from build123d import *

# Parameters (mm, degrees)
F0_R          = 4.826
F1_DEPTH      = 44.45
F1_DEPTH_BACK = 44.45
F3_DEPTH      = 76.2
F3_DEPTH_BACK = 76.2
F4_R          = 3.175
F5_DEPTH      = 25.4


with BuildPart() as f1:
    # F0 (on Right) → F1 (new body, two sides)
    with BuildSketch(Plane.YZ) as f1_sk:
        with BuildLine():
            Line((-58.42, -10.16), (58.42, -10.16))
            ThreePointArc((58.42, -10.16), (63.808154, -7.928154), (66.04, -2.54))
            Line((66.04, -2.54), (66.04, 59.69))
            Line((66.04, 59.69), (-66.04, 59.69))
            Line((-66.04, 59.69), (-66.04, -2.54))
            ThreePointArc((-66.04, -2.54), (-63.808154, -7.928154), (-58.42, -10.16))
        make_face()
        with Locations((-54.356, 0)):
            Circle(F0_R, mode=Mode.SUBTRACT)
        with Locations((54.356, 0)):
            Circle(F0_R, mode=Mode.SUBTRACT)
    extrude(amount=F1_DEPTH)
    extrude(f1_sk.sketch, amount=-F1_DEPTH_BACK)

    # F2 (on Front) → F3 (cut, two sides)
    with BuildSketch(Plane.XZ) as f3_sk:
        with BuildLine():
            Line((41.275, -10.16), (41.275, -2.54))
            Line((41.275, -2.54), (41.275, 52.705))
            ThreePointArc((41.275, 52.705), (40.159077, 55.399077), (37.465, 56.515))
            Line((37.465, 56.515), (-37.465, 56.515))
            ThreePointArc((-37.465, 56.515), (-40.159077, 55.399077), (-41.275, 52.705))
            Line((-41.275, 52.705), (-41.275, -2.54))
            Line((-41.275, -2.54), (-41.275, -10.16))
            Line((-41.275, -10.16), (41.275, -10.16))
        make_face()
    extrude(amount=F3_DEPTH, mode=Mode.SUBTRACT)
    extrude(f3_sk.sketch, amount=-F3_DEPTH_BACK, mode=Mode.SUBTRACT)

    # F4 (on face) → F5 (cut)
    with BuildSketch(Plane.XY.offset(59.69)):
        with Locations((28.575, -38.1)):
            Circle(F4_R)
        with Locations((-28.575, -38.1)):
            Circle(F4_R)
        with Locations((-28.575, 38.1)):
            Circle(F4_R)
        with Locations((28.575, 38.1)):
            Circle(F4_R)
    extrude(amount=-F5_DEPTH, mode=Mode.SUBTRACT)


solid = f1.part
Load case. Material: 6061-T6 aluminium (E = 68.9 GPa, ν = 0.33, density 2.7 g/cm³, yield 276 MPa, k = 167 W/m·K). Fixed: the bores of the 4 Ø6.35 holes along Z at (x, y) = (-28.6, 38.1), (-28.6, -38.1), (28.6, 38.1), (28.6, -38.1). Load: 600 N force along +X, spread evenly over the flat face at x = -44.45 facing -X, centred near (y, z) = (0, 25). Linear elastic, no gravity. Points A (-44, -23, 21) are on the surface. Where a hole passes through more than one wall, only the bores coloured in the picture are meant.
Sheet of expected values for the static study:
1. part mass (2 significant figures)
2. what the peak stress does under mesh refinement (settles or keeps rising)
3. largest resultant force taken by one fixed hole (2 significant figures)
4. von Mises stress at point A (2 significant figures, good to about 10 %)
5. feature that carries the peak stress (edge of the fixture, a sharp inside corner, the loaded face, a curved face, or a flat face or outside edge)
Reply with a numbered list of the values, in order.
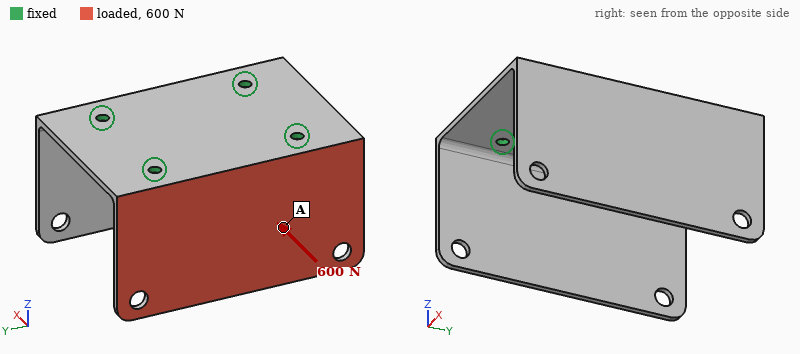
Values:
1. 250 g
2. keeps rising
3. 230 N
4. 16 MPa
5. edge of the fixture
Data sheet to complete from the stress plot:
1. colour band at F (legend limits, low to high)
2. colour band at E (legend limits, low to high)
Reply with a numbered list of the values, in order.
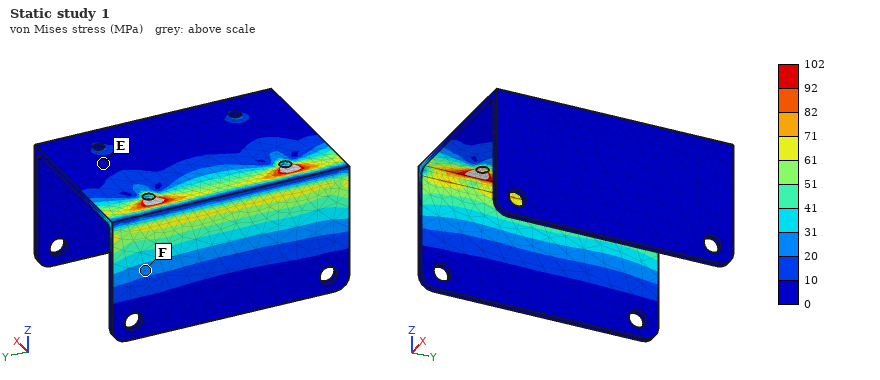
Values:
1. 20 to 31 MPa
2. 0 to 10 MPa
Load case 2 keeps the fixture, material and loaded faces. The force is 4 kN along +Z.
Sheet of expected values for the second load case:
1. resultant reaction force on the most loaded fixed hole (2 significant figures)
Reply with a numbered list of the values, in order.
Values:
1. 2.1 kN
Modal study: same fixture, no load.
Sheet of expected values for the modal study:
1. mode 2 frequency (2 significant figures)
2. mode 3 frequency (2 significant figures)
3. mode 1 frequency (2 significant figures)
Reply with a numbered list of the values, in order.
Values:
1. 460 Hz
2. 790 Hz
3. 450 Hz
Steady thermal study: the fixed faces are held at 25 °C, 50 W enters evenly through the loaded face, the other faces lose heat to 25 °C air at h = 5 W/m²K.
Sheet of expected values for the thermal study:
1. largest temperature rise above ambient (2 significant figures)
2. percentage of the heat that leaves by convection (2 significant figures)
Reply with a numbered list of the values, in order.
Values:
1. 38 K
2. 4.4 %
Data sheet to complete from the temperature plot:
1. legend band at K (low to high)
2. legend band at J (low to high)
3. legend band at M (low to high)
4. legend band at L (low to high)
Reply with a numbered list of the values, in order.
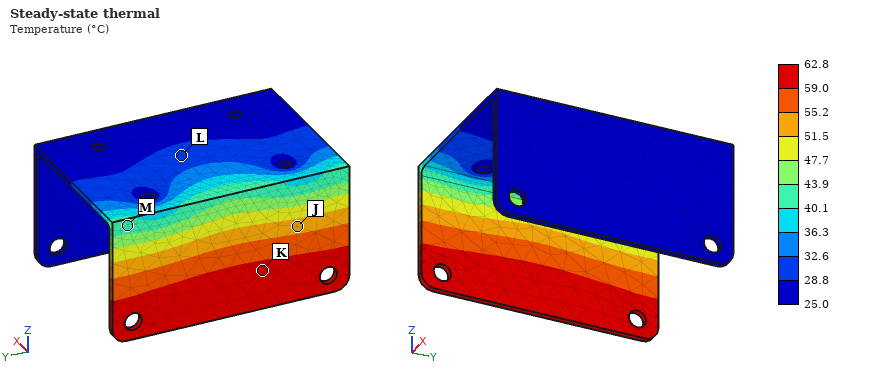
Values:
1. 59.0 to 62.8 °C
2. 51.5 to 55.2 °C
3. 40.1 to 43.9 °C
4. 28.8 to 32.6 °C
